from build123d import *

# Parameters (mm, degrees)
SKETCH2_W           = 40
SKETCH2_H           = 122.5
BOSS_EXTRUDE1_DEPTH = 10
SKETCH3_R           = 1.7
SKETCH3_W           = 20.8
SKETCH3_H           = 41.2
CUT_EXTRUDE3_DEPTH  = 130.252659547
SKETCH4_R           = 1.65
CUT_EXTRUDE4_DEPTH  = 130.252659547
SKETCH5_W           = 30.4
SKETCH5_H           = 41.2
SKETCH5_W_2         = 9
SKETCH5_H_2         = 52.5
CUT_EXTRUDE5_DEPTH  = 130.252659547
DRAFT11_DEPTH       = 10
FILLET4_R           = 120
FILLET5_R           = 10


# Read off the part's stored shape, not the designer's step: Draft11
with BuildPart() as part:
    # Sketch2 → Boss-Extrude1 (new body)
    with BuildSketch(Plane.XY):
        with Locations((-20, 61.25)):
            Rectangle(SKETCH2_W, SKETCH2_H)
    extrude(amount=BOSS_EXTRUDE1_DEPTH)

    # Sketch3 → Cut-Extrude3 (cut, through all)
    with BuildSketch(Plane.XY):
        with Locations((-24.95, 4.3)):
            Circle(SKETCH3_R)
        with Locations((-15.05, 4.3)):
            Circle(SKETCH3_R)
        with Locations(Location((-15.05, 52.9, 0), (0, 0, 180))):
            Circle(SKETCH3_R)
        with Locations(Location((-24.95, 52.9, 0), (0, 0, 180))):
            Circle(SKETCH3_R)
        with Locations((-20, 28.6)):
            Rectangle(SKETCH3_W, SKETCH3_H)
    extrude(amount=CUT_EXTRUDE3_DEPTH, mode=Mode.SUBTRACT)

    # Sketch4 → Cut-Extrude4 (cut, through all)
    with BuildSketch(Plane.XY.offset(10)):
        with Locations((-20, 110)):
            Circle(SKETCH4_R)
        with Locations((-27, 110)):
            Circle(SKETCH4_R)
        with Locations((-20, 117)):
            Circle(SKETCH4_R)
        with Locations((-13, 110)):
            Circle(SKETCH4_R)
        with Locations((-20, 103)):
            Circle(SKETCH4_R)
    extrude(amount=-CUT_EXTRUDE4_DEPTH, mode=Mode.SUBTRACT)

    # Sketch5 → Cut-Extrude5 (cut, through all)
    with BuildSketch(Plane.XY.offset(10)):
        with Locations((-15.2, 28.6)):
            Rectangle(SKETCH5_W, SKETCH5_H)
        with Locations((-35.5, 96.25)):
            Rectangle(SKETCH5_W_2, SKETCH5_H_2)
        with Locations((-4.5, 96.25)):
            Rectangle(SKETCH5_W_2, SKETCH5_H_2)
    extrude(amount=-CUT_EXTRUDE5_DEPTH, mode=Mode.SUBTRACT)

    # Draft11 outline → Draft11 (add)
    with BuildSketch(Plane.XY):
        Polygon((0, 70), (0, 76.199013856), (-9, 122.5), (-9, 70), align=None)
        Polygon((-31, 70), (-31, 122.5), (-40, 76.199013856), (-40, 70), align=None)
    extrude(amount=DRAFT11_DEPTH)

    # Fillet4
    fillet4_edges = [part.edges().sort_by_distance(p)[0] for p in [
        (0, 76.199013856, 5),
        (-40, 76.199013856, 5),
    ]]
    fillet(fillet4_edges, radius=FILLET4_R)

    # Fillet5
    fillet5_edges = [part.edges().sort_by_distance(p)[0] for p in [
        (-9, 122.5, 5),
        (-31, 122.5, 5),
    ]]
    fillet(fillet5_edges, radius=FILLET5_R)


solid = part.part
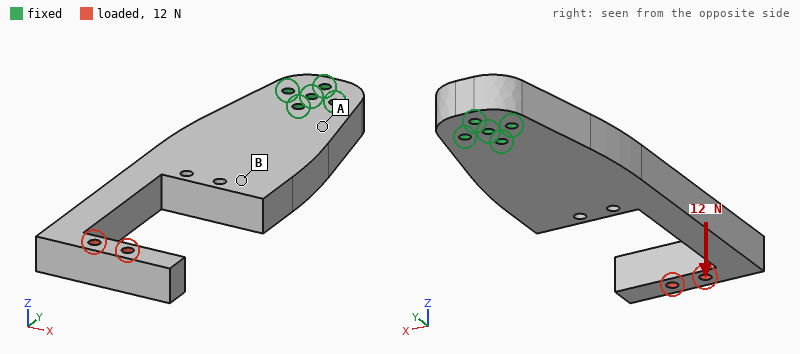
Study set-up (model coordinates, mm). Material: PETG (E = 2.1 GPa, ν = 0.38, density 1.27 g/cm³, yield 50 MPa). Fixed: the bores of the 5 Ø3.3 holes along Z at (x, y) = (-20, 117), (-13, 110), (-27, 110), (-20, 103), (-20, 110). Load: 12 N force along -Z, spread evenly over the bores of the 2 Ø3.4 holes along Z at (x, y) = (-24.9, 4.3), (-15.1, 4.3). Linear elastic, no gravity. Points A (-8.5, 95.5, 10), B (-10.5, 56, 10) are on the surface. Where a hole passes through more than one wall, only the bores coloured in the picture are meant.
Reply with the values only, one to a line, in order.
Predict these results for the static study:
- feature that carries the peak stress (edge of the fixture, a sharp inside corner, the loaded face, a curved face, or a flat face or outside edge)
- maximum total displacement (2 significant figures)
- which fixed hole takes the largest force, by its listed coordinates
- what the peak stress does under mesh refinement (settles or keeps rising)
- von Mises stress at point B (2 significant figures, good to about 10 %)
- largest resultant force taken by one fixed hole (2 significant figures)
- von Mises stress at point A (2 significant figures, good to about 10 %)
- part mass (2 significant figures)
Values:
edge of the fixture
1.4 mm
(-20, 103)
keeps rising
0.48 MPa
56 N
1.8 MPa
40 g
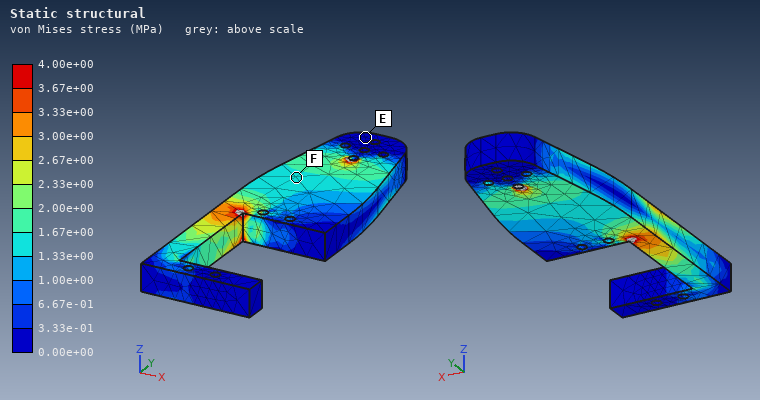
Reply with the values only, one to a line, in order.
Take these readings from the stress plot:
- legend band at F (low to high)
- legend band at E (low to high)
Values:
1.33e+00 to 1.67e+00 MPa
0.00e+00 to 3.33e-01 MPa
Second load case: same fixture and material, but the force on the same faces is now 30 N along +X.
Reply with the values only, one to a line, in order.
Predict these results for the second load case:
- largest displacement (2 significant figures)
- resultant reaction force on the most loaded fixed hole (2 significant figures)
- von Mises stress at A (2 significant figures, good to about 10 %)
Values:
1.5 mm
130 N
1.2 MPa
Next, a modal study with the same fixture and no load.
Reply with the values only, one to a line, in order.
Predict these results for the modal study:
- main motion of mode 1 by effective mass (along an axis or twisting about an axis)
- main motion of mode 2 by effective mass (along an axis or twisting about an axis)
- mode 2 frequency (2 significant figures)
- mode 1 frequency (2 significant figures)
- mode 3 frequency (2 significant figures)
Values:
along Z
along X
340 Hz
210 Hz
620 Hz
